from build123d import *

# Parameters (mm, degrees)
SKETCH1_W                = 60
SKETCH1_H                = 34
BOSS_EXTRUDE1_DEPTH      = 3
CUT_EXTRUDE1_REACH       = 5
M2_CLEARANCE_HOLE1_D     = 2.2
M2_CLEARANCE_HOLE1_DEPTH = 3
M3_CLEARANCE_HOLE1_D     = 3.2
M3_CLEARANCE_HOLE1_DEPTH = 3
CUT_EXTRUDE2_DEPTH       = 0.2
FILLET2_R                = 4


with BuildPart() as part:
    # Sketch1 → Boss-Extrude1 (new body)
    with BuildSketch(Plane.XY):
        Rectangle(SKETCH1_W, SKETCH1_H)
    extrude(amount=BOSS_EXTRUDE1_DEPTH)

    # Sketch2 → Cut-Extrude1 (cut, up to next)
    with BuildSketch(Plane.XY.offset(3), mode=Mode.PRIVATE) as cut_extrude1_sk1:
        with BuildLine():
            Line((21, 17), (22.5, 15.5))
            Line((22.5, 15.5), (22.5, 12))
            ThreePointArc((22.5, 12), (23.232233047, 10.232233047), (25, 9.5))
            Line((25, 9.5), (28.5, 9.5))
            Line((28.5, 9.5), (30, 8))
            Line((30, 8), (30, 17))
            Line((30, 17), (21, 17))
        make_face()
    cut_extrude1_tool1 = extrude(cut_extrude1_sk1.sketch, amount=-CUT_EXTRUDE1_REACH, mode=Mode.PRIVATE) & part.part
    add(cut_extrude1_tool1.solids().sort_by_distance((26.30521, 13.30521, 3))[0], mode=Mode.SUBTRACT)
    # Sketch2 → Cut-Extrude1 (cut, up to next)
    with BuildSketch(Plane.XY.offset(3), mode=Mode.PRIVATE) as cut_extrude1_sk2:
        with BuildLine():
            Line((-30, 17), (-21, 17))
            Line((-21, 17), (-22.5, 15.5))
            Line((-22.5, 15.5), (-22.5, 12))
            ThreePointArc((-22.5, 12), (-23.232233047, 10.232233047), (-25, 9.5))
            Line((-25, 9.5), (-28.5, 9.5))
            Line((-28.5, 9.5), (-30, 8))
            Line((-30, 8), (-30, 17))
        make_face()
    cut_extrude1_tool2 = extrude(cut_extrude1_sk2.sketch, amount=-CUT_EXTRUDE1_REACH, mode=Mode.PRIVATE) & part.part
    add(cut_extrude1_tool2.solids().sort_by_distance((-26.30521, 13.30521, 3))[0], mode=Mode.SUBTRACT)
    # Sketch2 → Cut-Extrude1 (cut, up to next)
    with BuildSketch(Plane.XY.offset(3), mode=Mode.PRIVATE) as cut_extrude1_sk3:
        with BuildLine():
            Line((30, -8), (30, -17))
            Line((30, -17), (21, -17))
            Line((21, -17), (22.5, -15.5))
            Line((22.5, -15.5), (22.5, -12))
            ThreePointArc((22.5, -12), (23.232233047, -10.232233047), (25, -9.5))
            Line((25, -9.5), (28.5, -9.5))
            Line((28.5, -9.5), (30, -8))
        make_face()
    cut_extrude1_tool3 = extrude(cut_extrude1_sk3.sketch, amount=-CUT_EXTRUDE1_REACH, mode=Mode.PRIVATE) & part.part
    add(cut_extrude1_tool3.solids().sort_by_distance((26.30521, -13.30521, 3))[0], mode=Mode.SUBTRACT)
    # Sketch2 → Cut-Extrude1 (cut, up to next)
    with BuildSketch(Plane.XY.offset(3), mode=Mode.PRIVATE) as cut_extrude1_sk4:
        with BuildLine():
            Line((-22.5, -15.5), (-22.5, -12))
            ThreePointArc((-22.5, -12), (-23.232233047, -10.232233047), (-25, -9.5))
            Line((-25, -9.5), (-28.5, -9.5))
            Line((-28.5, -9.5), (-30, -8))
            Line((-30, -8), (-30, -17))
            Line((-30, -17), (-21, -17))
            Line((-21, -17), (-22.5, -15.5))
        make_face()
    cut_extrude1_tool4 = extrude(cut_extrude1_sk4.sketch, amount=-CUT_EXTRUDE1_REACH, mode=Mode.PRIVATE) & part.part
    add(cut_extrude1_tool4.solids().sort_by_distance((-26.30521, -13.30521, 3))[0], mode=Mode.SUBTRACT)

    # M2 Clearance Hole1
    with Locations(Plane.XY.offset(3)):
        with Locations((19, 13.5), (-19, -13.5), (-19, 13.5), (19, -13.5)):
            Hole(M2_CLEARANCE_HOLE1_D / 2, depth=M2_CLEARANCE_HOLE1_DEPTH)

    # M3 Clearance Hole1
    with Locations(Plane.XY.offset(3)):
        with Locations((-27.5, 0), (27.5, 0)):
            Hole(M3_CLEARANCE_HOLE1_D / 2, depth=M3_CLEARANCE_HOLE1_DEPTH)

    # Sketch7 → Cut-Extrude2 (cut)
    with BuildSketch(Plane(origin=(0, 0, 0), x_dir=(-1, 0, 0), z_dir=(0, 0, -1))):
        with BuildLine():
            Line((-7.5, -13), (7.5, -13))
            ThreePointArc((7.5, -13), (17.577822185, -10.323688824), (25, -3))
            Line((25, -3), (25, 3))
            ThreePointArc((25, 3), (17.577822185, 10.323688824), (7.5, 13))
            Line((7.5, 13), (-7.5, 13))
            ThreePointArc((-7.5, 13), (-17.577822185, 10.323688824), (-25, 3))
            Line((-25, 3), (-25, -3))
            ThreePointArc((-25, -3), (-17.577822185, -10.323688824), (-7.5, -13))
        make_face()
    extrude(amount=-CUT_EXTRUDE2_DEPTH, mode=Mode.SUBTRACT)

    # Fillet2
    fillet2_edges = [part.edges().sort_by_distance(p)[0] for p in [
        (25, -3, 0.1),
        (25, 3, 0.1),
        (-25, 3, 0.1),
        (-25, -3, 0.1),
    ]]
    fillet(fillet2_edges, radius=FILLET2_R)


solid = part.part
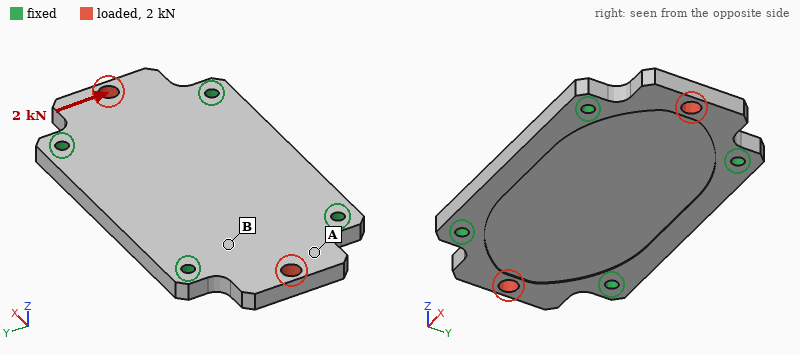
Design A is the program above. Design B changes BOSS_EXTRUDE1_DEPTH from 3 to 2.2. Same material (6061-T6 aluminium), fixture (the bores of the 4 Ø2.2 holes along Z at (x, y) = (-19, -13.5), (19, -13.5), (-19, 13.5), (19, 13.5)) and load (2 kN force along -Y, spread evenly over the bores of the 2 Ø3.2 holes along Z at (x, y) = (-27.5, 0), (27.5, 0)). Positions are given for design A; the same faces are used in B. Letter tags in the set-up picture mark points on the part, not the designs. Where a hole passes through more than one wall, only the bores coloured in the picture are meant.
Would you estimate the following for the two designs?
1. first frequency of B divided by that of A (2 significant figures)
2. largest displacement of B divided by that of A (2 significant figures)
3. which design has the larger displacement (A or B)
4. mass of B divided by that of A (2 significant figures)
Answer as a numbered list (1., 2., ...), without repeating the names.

1. 0.76
2. 1.4
3. B
4. 0.72
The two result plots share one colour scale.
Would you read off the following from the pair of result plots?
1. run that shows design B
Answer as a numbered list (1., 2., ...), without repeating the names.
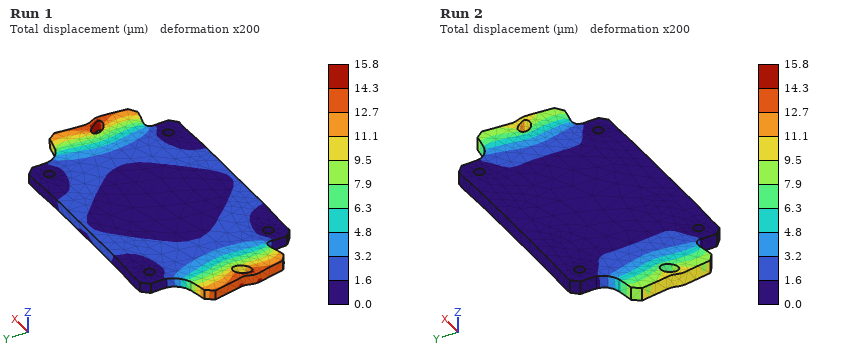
1. Run 1
